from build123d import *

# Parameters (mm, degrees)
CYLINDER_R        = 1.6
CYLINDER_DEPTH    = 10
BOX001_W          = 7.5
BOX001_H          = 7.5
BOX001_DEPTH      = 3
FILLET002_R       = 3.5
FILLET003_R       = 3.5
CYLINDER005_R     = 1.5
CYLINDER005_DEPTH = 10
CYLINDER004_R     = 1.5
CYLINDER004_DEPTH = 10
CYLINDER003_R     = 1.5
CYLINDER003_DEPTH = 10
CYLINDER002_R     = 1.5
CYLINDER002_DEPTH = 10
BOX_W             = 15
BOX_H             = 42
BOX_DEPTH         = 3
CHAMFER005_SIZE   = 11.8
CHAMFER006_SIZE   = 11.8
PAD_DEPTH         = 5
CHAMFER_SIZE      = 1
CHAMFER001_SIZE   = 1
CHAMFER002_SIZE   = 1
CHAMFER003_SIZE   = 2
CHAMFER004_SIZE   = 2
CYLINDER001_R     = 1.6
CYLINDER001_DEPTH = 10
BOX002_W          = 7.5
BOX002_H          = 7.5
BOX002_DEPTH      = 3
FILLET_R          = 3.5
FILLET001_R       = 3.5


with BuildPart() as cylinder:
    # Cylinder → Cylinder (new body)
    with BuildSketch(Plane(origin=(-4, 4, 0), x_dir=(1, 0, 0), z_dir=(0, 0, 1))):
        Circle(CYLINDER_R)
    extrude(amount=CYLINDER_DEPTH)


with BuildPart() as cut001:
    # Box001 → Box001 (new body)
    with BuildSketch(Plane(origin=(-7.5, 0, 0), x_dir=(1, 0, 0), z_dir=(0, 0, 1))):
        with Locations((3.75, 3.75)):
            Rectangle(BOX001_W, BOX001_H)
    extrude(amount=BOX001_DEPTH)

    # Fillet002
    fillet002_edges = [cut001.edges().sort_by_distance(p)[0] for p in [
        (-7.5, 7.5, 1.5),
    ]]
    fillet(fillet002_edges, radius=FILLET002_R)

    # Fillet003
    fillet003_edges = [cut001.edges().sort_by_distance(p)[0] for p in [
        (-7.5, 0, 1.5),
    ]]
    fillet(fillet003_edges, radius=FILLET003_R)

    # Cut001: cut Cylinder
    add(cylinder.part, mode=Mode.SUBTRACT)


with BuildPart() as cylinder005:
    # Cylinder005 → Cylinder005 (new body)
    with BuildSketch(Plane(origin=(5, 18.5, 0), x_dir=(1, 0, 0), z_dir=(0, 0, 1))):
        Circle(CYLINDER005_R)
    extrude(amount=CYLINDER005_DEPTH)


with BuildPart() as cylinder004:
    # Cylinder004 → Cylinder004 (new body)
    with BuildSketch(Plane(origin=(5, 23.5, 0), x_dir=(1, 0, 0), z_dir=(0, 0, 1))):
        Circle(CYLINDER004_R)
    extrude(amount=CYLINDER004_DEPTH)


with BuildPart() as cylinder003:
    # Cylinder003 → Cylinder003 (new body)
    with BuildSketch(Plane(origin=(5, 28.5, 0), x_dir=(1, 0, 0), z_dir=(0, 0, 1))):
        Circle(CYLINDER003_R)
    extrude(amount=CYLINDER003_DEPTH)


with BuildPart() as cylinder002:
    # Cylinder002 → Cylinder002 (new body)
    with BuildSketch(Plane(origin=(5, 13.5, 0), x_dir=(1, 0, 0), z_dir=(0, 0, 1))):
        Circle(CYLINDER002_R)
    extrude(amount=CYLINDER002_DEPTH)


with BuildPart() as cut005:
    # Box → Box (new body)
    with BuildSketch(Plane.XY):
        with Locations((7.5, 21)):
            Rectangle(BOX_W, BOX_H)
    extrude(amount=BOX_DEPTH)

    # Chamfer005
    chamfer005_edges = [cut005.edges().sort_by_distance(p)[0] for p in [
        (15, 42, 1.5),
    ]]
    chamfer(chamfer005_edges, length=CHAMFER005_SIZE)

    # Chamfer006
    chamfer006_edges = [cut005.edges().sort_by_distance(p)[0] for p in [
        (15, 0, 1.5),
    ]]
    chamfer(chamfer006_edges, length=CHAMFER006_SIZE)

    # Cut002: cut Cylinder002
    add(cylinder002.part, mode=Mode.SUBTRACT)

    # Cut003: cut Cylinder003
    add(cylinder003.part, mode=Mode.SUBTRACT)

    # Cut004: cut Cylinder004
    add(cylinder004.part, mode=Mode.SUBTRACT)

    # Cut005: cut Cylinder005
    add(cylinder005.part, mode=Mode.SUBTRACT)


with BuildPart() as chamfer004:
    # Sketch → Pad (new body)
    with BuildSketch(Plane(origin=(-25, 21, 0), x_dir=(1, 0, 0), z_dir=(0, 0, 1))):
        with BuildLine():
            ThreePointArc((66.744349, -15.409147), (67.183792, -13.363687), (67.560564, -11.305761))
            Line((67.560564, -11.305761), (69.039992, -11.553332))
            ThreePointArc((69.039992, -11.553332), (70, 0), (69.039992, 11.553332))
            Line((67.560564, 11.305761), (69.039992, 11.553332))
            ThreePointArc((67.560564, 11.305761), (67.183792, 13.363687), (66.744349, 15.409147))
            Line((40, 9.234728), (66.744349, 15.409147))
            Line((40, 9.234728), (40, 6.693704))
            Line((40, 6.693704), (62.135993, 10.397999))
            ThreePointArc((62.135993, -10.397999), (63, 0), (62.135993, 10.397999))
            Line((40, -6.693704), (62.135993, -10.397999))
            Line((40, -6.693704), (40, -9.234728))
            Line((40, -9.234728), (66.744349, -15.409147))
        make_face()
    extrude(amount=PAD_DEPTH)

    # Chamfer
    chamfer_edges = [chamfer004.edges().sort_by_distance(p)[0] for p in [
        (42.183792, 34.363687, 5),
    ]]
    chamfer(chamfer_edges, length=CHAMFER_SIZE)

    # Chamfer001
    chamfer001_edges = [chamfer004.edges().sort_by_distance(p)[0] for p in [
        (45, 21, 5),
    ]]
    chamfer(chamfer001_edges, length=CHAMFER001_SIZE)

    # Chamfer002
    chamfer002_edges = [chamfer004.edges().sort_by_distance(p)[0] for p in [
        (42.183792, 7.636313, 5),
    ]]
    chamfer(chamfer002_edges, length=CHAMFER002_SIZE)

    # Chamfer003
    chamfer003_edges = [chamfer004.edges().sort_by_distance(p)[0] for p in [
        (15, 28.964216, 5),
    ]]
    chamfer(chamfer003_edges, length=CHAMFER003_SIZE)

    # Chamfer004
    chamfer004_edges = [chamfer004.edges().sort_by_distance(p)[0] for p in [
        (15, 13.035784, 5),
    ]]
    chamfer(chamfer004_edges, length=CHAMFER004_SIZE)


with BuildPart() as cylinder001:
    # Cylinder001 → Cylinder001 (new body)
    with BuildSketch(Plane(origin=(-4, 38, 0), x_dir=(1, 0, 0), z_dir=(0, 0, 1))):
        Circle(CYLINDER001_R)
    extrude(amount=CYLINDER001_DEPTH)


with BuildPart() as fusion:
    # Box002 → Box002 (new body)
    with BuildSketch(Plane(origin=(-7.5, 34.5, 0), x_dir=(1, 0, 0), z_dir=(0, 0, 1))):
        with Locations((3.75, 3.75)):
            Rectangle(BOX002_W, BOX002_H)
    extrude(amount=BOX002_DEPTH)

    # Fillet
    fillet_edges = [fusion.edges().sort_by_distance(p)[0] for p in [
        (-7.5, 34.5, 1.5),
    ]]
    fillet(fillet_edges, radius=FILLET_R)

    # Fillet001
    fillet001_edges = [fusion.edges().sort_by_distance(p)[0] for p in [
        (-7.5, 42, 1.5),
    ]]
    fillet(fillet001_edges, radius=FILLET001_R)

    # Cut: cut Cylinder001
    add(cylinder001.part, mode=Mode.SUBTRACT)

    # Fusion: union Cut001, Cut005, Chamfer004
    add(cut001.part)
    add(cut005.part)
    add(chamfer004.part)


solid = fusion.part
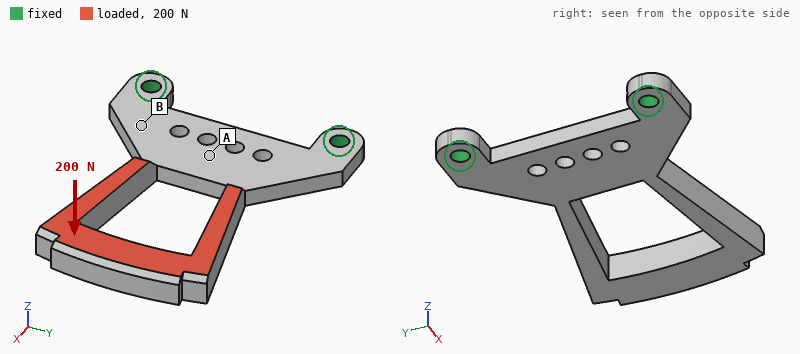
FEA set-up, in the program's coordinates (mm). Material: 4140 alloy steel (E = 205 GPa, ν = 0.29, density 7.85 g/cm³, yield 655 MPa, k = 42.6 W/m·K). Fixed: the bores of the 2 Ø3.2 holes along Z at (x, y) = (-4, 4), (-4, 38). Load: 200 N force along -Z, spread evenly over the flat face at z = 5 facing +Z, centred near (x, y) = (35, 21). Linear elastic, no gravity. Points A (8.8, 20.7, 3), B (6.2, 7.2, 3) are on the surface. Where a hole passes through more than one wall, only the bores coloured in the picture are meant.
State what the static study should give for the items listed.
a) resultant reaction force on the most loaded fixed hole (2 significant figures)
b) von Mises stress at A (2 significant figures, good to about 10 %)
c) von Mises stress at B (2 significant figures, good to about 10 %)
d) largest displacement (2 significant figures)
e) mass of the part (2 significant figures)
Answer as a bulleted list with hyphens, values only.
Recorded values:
- 100 N
- 79 MPa
- 210 MPa
- 0.80 mm
- 26 g
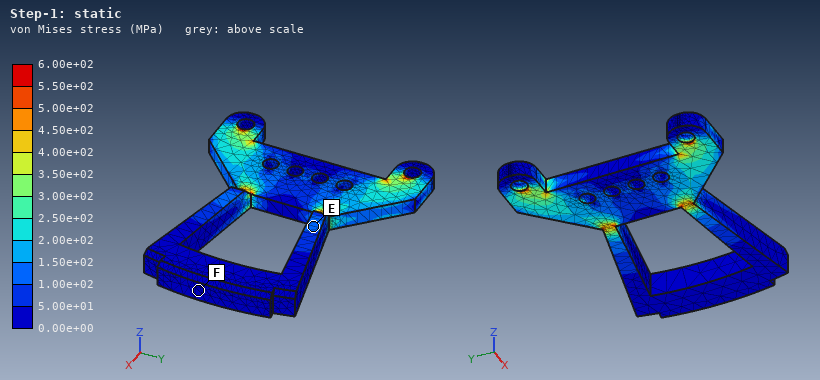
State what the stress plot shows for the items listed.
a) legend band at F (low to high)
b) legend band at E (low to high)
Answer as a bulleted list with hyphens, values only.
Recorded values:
- 0.00e+00 to 5.00e+01 MPa
- 1.00e+02 to 1.50e+02 MPa
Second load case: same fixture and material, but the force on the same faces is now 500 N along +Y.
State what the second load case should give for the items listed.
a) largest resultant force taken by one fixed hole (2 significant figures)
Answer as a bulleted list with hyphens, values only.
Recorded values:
- 590 N
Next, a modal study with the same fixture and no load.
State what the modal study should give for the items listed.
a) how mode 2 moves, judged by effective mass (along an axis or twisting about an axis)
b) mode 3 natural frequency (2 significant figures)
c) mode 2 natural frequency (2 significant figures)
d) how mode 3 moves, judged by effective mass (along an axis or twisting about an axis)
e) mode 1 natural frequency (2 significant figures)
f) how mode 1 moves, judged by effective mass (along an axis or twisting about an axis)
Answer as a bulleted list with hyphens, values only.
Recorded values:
- along Y
- 2800 Hz
- 2100 Hz
- twisting about X
- 770 Hz
- along Z
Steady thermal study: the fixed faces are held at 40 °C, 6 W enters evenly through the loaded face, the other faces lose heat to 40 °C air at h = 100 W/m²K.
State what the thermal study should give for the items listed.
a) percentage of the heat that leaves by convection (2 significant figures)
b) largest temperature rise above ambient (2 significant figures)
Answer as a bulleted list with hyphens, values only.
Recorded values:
- 83 %
- 45 K
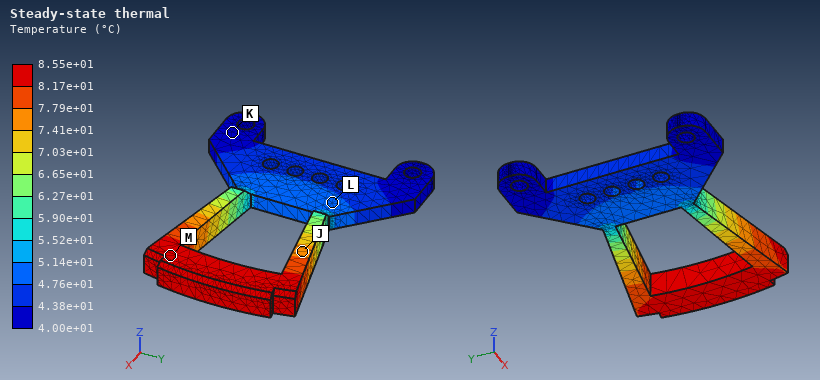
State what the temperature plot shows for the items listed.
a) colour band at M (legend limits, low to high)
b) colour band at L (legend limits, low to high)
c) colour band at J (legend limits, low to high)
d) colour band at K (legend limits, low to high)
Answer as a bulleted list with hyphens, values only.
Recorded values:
- 8.17e+01 to 8.55e+01 °C
- 4.76e+01 to 5.14e+01 °C
- 7.41e+01 to 7.79e+01 °C
- 4.00e+01 to 4.38e+01 °C
